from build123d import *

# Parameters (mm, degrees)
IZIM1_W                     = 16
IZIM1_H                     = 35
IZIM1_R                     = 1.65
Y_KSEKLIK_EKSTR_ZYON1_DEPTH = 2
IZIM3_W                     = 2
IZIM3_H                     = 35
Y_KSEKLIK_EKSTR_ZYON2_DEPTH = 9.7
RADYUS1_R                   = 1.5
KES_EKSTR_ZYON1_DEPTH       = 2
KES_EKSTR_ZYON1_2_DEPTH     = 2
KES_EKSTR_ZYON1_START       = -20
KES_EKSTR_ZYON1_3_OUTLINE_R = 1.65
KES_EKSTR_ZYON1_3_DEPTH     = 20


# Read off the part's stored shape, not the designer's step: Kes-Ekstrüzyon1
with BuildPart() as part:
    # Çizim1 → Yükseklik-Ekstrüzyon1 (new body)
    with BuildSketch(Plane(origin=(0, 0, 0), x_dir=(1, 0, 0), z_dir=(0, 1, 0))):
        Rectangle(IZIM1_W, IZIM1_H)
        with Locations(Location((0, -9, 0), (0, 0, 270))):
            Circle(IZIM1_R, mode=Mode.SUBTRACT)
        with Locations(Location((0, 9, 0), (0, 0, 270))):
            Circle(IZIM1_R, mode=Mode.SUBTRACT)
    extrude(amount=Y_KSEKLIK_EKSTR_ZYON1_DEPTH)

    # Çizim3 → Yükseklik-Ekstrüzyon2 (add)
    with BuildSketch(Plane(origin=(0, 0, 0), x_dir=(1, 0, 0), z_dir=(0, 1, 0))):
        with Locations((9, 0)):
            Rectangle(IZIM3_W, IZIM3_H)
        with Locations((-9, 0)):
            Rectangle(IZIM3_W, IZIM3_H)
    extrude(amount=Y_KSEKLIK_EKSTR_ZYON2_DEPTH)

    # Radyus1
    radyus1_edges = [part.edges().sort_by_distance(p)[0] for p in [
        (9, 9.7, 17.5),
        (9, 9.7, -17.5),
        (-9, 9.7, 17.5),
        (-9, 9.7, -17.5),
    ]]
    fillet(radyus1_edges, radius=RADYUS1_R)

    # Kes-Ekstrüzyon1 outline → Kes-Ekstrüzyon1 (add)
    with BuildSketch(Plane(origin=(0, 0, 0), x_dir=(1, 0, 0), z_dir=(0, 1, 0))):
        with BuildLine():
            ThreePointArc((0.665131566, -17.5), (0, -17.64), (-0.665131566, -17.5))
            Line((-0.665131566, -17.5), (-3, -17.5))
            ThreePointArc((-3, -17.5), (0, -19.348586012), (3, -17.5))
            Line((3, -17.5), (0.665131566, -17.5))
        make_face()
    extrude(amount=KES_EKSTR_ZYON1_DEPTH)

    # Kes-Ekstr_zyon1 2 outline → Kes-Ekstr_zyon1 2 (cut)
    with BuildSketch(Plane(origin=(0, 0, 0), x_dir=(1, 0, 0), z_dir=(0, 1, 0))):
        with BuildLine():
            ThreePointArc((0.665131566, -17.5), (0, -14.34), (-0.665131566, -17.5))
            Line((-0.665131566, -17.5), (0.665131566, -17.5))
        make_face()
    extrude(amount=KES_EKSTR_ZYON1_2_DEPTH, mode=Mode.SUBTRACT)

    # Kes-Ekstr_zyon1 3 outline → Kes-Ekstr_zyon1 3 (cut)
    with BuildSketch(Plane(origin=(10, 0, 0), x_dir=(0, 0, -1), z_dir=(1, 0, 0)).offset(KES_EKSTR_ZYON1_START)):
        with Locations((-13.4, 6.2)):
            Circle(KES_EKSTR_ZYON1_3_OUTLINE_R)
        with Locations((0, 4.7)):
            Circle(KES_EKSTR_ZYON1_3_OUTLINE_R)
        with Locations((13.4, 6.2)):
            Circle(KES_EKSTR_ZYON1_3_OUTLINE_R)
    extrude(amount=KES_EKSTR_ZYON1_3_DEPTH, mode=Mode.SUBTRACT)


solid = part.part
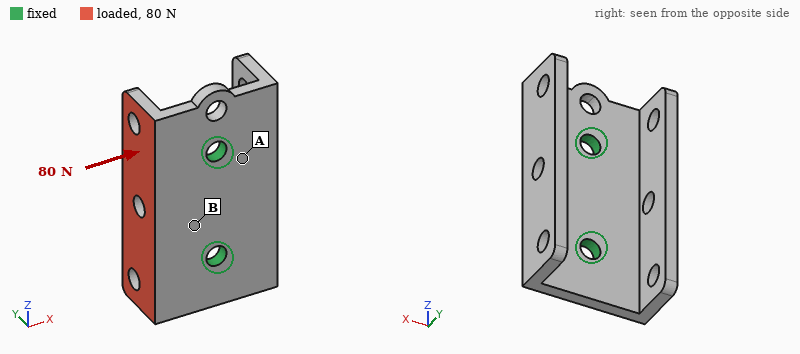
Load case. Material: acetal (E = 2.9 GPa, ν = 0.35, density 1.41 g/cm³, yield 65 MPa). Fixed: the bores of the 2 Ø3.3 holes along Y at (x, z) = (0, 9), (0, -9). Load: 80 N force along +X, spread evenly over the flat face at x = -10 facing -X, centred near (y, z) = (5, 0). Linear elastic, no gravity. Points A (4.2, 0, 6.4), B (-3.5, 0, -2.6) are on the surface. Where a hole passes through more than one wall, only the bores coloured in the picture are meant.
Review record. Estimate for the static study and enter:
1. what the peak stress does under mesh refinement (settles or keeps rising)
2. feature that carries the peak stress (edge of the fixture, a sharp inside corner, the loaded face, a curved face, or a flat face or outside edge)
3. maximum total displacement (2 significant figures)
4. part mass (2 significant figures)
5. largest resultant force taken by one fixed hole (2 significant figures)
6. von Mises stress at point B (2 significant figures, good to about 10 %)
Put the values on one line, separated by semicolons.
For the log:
keeps rising; edge of the fixture; 0.45 mm; 3.3 g; 40 N; 9.2 MPa
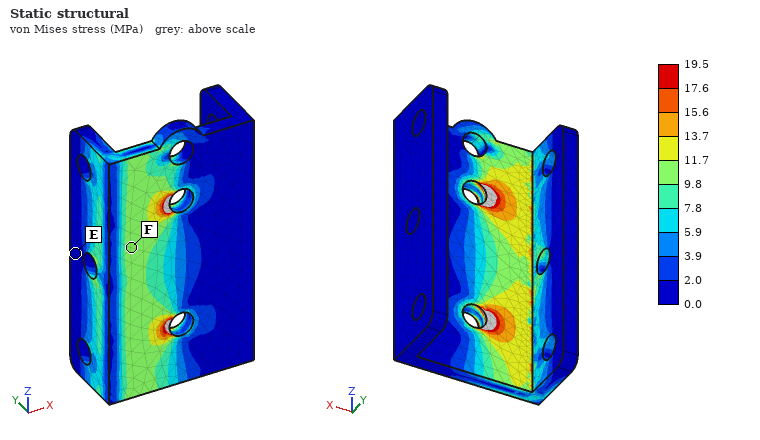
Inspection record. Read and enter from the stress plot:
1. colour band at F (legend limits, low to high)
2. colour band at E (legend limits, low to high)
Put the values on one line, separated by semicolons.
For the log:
9.8 to 11.7 MPa; 0.0 to 2.0 MPa
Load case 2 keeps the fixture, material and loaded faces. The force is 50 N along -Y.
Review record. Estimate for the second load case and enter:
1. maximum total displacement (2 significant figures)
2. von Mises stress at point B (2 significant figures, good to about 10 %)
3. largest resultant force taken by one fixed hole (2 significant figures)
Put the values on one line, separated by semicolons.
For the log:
0.39 mm; 9.5 MPa; 25 N
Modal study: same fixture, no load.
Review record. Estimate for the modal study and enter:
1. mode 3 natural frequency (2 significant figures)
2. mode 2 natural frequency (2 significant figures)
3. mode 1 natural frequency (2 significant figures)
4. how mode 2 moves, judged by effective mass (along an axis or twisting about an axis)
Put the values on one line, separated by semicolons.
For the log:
2600 Hz; 2300 Hz; 2000 Hz; along Y
